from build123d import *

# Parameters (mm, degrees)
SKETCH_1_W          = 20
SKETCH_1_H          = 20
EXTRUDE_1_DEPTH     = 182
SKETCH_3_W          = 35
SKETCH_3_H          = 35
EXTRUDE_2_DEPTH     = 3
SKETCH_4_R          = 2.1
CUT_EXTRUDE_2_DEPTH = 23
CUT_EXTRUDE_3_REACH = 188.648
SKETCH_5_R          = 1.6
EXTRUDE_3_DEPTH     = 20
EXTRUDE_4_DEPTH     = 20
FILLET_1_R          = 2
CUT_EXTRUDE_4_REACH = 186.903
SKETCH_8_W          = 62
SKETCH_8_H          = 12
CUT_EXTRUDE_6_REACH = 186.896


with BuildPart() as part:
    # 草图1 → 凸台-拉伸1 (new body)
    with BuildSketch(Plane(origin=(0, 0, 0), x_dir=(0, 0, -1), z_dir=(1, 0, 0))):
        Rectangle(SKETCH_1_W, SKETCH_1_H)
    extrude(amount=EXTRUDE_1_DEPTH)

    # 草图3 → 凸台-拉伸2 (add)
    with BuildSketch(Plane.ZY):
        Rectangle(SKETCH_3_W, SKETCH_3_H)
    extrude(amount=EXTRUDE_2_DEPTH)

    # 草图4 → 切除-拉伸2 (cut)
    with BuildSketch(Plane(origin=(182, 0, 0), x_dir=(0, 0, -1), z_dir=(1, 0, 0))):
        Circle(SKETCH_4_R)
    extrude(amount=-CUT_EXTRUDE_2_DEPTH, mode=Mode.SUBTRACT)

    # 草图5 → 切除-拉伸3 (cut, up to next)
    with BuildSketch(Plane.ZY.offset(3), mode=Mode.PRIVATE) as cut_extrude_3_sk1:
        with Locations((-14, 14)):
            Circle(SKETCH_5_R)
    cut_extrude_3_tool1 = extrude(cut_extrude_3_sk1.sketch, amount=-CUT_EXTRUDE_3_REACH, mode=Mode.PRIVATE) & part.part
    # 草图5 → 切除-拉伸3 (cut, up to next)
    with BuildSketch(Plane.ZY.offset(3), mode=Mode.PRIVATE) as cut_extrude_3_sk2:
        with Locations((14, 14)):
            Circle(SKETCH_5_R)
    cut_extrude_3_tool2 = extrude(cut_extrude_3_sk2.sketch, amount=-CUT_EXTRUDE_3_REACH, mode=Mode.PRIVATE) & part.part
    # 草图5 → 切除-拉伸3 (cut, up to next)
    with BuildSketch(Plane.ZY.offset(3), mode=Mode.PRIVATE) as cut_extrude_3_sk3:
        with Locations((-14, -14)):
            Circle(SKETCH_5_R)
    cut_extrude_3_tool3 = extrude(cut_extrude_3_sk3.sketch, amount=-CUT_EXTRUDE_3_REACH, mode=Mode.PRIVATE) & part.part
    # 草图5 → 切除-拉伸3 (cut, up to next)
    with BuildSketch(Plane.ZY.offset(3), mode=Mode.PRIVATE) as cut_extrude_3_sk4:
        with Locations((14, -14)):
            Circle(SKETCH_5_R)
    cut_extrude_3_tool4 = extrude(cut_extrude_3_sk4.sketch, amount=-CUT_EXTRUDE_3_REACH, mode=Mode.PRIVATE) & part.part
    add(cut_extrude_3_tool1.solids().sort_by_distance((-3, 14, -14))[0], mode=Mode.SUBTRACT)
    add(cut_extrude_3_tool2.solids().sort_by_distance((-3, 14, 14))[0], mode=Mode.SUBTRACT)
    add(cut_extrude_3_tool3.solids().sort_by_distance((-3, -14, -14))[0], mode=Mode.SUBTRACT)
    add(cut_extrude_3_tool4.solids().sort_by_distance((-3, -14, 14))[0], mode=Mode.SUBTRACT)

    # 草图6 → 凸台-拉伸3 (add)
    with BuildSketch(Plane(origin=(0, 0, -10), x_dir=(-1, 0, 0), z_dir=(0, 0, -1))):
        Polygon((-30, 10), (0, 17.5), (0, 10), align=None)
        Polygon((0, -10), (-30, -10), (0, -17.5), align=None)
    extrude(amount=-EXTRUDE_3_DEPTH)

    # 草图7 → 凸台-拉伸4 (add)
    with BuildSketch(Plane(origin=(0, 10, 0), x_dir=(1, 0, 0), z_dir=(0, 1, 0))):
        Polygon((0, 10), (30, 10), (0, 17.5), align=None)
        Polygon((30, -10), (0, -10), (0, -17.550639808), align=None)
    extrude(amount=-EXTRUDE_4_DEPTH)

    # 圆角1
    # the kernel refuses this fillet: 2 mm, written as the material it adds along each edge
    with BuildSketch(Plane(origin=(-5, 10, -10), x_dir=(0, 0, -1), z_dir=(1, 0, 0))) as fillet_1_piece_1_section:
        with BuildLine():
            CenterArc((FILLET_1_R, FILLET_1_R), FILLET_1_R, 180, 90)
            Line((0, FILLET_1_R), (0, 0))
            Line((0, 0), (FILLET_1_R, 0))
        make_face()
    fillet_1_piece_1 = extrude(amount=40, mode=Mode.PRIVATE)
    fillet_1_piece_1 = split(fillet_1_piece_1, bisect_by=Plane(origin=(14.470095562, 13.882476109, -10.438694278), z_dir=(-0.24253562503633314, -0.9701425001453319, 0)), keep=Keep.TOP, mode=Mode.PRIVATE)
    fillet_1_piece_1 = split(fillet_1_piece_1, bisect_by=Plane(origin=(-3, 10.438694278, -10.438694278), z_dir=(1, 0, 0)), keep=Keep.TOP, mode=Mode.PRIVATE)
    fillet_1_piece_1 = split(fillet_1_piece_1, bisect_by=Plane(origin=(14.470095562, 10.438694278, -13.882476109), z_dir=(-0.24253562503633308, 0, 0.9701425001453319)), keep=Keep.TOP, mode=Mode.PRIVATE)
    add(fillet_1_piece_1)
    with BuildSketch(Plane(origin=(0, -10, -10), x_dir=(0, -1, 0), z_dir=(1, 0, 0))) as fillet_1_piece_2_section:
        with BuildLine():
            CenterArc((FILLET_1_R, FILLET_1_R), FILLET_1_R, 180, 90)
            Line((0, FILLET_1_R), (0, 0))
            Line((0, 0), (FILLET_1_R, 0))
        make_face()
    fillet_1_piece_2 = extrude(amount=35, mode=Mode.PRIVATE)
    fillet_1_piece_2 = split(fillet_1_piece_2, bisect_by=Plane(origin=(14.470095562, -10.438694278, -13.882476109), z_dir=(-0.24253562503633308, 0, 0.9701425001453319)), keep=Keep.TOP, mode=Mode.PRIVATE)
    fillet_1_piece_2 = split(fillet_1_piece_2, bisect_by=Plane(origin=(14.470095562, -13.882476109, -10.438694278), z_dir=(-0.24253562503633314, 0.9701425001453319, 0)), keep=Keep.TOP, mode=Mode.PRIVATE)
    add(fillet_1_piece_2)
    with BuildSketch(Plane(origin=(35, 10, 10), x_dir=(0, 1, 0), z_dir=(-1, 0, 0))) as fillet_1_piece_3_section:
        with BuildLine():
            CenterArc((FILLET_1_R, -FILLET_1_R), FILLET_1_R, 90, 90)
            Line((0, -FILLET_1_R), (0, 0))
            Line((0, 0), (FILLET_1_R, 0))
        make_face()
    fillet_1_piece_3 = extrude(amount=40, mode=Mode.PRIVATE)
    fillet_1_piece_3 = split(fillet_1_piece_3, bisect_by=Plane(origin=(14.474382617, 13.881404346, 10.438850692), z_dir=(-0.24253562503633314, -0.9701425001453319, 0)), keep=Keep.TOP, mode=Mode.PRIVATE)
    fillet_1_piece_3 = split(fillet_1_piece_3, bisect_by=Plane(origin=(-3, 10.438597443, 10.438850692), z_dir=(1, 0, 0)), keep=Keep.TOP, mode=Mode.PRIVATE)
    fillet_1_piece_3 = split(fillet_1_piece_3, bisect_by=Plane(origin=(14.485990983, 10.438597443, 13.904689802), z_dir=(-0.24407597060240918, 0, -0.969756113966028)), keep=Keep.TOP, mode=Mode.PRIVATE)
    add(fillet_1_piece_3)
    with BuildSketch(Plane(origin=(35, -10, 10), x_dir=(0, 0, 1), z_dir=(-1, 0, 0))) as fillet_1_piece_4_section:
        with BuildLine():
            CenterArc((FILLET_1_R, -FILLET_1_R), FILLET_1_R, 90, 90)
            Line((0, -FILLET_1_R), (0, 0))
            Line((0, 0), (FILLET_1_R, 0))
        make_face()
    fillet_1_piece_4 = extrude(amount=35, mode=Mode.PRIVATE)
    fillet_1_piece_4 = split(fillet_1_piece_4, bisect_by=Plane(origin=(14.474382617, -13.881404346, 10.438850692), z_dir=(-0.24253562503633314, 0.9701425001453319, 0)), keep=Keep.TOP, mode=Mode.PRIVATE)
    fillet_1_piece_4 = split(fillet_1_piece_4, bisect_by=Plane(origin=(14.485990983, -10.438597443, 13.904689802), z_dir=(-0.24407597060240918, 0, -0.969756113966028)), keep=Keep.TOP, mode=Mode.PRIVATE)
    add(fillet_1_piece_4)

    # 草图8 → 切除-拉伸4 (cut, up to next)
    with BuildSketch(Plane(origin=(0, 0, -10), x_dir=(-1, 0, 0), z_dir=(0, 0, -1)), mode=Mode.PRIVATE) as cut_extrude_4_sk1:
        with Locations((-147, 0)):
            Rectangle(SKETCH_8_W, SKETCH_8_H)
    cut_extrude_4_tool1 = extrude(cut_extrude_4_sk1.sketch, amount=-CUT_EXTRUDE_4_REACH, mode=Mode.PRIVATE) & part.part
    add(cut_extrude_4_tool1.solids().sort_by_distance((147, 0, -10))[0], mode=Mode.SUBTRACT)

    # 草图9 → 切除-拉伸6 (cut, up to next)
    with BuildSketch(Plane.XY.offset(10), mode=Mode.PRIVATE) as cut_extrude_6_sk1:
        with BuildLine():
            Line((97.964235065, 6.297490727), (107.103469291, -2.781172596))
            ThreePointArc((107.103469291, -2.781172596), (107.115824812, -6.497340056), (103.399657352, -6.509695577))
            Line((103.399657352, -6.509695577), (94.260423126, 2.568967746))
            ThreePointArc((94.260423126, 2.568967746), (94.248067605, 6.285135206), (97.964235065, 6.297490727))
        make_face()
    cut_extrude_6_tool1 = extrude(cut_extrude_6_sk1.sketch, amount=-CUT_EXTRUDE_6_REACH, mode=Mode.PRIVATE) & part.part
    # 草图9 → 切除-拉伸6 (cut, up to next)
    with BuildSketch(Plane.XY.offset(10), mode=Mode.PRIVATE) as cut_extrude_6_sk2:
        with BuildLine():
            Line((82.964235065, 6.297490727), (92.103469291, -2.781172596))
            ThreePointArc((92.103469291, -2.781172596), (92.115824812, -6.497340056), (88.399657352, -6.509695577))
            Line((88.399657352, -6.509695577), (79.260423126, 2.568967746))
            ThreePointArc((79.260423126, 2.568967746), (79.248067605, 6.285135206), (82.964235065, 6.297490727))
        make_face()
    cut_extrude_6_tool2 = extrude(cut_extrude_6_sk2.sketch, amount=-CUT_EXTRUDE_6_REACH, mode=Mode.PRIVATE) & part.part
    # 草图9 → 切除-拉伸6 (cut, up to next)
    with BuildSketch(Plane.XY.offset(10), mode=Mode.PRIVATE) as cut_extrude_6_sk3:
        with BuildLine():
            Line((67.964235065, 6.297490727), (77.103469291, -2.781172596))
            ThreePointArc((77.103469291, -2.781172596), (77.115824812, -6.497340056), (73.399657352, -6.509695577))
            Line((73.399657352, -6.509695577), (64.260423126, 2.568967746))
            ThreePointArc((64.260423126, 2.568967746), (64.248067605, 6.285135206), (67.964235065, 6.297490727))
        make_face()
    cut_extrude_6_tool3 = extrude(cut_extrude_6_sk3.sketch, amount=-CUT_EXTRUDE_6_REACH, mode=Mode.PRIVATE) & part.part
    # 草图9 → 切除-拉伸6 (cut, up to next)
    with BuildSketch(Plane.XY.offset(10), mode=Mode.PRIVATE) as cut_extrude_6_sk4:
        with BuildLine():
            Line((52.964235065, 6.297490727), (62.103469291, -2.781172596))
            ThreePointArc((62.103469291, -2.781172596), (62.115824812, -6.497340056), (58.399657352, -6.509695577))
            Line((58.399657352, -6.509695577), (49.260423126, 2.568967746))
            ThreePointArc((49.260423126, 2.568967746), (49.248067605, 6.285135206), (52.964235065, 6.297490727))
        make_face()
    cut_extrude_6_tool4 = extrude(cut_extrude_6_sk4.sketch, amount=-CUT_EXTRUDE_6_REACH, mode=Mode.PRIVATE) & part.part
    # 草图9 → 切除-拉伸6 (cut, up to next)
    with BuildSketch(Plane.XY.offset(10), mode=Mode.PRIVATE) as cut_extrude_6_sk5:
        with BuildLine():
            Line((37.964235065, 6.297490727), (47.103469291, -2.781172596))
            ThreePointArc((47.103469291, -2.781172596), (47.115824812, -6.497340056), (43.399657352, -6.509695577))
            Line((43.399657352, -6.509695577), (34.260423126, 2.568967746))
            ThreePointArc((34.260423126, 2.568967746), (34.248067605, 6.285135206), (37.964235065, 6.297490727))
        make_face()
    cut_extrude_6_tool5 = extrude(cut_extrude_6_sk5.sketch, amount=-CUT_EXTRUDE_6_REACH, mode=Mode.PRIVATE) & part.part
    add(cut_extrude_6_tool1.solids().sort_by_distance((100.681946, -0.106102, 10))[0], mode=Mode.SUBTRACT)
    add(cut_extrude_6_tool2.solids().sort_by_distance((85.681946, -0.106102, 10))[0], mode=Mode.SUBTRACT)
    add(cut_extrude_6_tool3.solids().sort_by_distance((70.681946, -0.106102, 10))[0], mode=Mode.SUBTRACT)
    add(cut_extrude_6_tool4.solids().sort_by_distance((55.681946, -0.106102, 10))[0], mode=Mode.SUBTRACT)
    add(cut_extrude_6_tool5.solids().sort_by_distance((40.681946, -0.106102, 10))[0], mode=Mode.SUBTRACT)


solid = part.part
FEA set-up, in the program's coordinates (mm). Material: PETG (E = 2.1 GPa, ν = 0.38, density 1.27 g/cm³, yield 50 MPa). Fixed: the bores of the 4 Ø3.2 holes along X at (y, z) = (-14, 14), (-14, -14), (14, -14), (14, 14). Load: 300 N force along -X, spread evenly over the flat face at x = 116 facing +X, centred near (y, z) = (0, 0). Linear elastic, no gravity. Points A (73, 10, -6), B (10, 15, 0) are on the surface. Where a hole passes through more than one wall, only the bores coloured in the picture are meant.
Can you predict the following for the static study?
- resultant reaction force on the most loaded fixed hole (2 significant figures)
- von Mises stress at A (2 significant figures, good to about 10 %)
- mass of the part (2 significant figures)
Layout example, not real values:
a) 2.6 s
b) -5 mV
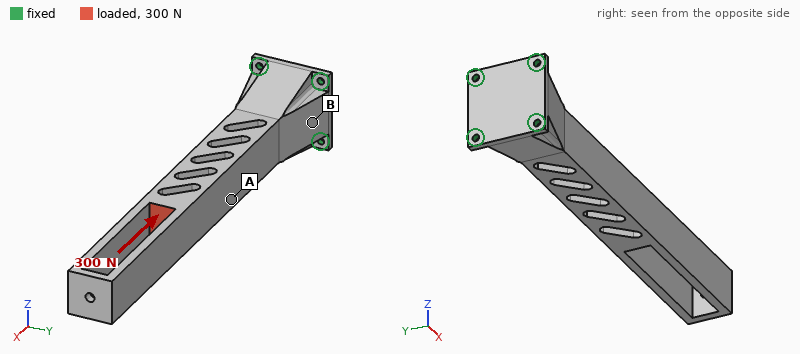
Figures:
a) 81 N
b) 2.3 MPa
c) 78 g
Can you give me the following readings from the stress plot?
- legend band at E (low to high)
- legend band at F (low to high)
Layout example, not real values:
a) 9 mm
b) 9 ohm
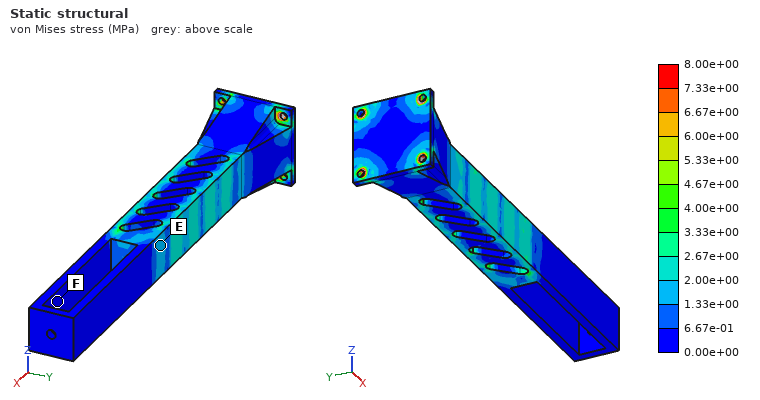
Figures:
a) 1.33e+00 to 2.00e+00 MPa
b) 0.00e+00 to 6.67e-01 MPa
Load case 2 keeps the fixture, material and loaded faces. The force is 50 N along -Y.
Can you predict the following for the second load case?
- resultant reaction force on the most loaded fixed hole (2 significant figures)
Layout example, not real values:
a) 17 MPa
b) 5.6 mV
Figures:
a) 120 N
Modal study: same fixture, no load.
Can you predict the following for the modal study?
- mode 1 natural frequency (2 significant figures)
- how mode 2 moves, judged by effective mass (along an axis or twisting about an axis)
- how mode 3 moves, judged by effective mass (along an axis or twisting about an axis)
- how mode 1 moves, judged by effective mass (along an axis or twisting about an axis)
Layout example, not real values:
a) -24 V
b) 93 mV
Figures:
a) 130 Hz
b) along Y
c) along Y
d) along Z
